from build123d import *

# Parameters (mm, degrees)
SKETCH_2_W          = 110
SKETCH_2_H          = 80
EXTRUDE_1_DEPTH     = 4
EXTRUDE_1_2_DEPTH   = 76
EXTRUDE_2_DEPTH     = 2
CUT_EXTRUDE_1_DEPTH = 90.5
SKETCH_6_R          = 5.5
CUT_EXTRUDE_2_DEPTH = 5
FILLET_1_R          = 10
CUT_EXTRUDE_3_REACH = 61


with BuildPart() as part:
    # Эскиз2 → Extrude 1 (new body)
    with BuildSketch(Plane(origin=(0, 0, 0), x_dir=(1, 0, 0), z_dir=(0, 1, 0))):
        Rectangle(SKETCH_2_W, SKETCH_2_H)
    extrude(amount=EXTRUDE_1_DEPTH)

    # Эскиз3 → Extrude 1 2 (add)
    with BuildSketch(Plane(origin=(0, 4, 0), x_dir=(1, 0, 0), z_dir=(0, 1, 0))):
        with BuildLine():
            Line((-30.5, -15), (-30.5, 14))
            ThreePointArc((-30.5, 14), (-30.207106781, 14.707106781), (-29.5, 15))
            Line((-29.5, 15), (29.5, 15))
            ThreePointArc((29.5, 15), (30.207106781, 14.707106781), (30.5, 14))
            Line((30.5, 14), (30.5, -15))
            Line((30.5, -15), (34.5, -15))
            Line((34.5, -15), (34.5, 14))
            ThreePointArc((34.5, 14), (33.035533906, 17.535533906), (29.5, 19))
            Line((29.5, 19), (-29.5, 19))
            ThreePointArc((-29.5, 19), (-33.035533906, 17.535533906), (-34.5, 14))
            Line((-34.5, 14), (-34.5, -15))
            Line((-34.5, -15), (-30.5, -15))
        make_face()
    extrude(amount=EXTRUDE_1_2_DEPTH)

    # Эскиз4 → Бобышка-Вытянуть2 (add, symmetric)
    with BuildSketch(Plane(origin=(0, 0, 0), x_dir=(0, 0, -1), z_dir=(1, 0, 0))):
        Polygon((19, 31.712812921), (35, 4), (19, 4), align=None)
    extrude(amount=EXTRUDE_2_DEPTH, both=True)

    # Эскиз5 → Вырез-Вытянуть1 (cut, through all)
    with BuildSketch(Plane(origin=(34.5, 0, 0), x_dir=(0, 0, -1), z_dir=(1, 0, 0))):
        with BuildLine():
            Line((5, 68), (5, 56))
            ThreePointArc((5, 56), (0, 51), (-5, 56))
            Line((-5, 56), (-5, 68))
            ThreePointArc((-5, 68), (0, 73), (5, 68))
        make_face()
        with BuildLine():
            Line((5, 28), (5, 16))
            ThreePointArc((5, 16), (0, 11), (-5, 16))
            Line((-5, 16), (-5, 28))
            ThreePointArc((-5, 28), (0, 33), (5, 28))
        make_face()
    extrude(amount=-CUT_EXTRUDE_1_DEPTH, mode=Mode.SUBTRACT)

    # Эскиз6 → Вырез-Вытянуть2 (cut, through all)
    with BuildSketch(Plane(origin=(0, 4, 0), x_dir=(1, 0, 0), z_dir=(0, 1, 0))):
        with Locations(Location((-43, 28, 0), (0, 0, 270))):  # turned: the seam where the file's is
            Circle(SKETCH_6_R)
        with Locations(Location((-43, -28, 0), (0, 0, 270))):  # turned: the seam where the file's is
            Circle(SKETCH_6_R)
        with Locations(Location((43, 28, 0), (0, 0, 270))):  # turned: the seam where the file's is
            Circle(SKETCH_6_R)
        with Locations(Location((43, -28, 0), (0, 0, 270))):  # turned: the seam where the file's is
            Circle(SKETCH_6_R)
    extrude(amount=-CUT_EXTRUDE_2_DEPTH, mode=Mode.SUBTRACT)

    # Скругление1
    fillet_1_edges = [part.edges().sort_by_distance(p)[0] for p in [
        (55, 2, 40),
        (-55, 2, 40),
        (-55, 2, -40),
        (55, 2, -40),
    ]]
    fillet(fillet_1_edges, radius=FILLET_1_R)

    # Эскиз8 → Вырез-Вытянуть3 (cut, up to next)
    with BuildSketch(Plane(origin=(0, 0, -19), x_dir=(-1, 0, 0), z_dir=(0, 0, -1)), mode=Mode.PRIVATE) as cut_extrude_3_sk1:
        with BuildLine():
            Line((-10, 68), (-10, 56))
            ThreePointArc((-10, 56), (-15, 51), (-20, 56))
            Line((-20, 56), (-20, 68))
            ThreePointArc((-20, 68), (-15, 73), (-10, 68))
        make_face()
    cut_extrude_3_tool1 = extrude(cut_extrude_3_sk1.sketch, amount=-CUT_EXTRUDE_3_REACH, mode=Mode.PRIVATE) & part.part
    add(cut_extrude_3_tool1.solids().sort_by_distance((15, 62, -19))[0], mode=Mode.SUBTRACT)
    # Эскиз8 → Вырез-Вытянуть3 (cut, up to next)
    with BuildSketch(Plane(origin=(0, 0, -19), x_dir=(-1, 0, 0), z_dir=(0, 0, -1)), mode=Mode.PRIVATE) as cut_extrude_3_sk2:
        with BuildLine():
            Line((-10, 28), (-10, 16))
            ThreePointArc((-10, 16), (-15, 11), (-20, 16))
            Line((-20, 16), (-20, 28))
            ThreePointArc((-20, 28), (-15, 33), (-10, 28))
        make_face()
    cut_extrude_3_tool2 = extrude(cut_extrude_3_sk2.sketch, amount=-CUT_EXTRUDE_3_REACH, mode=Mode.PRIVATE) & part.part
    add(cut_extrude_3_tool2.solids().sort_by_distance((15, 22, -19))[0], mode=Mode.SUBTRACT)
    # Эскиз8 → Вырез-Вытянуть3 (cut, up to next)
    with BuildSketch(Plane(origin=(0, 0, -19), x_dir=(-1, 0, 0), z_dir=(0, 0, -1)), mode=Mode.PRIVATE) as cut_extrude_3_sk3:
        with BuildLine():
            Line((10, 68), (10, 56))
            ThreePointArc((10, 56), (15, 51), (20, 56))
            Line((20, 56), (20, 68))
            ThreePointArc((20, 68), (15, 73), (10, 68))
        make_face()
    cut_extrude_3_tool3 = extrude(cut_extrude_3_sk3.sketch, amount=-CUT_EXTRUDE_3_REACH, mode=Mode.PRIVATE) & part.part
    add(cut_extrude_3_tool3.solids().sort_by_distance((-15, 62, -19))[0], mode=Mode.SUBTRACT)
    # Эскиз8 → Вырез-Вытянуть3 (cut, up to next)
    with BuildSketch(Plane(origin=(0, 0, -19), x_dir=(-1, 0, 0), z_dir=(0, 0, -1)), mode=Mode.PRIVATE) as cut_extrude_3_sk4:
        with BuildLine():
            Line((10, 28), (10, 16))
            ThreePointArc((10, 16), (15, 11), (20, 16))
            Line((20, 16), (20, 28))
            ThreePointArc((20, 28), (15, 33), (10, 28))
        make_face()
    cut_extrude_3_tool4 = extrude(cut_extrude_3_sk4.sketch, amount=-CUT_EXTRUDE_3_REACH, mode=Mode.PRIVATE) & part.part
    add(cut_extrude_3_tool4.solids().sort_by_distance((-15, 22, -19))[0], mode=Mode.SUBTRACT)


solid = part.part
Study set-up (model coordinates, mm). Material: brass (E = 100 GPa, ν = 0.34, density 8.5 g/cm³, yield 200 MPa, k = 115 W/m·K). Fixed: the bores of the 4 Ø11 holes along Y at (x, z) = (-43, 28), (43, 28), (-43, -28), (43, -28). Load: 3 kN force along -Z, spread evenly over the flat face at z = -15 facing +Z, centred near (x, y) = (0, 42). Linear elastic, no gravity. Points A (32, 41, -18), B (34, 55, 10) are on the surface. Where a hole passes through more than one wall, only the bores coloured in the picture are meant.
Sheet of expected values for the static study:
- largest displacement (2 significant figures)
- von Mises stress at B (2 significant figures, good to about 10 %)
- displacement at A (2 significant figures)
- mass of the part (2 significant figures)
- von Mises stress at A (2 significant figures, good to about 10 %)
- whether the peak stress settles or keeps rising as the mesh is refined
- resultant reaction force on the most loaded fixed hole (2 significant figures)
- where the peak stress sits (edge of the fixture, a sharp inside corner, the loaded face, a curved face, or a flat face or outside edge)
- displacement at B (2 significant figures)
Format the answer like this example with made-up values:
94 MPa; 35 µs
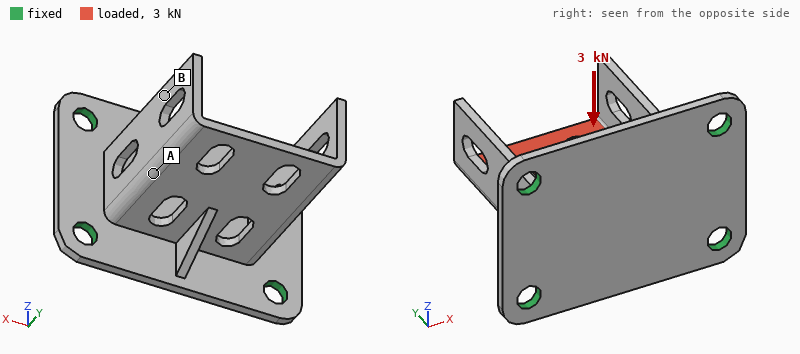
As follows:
0.46 mm; 16 MPa; 0.11 mm; 560 g; 41 MPa; keeps rising; 1.6 kN; edge of the fixture; 0.22 mm
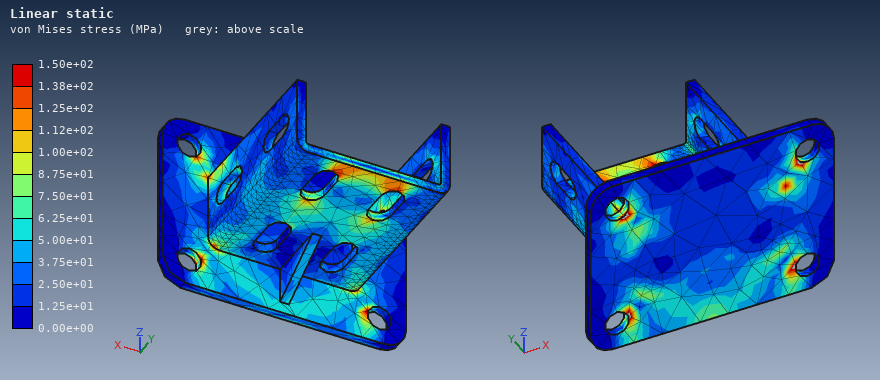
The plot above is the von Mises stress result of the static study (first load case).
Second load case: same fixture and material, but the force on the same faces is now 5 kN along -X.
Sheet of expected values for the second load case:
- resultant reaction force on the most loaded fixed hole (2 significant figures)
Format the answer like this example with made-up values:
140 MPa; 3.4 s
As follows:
3.2 kN
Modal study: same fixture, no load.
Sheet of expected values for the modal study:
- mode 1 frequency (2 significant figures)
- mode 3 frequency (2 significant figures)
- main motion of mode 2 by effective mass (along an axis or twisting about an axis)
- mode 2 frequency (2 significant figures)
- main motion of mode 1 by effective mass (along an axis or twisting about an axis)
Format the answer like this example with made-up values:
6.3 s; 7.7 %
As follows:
1100 Hz; 1500 Hz; along X; 1200 Hz; along Z
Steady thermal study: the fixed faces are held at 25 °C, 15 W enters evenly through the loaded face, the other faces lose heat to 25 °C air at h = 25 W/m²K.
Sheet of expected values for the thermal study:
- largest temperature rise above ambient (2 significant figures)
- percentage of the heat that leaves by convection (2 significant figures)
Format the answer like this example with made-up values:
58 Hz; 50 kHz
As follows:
15 K; 30 %
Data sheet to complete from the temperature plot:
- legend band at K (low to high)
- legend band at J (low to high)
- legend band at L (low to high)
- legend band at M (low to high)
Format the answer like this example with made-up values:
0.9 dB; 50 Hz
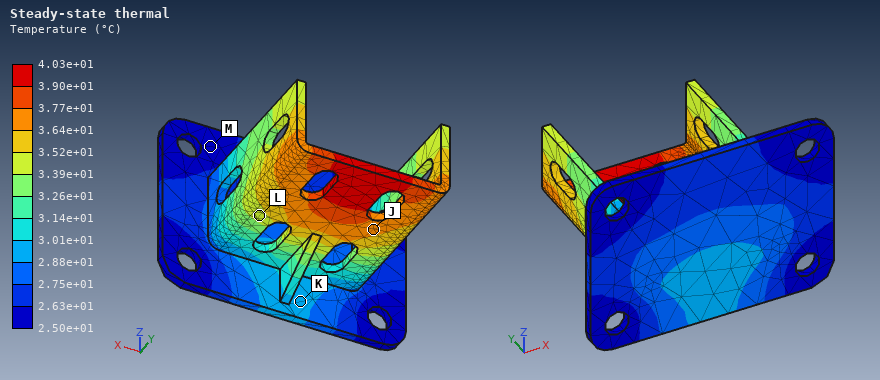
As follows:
2.88e+01 to 3.01e+01 °C; 3.64e+01 to 3.77e+01 °C; 3.39e+01 to 3.52e+01 °C; 2.50e+01 to 2.63e+01 °C
